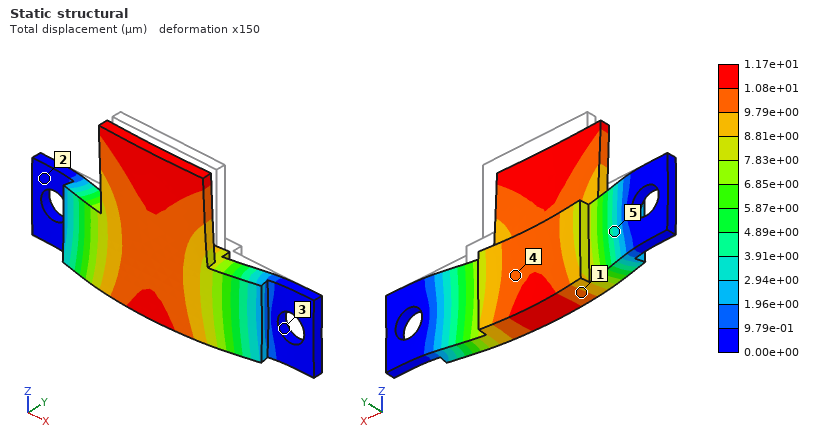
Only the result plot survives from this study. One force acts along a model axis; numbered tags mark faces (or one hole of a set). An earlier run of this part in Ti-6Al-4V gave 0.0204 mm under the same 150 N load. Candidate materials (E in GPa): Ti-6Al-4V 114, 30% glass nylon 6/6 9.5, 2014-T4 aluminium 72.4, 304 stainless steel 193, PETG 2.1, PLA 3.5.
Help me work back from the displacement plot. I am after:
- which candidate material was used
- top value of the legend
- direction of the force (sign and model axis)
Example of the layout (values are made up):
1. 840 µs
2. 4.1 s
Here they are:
1. 304 stainless steel
2. 1.17e+01 µm
3. -Y
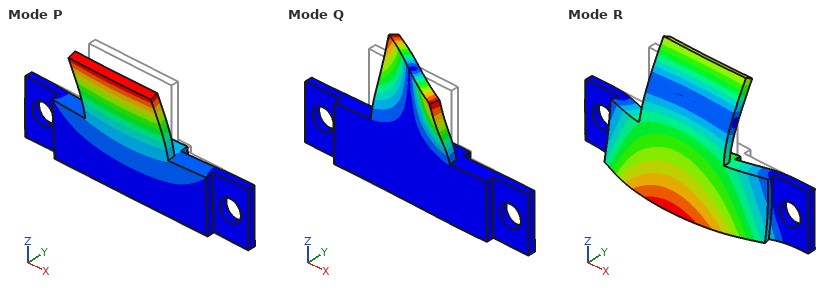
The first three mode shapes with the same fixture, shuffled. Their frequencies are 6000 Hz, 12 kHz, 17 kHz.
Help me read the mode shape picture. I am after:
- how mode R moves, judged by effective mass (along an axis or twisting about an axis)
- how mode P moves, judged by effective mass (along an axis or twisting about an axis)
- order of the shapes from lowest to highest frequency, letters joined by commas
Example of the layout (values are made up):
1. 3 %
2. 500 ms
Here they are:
1. along Y
2. along Y
3. P, R, Q
